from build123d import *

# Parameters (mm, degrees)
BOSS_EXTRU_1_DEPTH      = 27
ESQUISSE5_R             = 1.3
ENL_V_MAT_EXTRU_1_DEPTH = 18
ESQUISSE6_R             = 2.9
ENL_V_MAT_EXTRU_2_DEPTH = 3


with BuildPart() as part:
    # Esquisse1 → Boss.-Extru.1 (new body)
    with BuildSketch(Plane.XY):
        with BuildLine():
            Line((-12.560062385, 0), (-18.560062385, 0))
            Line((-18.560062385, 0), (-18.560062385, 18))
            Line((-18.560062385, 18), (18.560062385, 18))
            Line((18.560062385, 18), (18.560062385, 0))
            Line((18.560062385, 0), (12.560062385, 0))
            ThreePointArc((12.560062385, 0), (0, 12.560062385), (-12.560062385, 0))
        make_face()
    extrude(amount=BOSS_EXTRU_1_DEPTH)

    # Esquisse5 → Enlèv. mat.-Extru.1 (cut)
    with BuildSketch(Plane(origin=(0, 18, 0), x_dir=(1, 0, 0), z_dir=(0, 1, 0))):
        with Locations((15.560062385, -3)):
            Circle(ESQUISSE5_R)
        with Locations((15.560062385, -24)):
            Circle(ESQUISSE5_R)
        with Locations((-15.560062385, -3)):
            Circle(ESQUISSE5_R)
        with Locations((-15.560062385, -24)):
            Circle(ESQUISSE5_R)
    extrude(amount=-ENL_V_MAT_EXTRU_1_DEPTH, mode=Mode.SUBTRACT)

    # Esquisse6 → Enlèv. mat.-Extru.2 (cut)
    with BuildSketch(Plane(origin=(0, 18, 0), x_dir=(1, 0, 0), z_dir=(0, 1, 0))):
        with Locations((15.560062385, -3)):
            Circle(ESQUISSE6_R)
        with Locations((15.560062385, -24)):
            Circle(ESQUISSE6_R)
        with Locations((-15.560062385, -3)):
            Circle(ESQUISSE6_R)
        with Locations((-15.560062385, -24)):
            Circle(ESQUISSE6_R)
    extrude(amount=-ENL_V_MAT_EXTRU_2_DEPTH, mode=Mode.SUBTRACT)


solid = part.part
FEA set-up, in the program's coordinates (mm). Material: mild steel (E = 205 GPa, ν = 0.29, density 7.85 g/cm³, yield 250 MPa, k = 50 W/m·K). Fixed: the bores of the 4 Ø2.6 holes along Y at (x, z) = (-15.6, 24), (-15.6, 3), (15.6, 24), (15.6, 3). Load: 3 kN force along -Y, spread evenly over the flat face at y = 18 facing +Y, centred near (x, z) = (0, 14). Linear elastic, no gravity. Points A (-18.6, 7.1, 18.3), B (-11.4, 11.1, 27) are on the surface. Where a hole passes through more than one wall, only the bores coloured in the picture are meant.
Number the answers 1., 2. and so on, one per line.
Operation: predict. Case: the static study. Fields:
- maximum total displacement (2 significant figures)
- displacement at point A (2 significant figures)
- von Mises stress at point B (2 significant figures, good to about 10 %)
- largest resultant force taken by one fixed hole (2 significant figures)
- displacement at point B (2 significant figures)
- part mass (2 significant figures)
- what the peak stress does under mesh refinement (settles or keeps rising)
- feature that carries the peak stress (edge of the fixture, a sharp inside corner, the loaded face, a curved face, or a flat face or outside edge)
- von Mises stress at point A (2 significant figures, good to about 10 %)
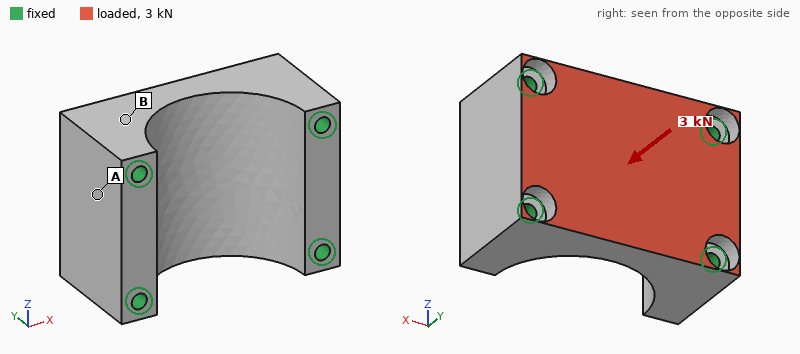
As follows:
1. 1.4 µm
2. 0.26 µm
3. 9.0 MPa
4. 870 N
5. 0.31 µm
6. 84 g
7. keeps rising
8. edge of the fixture
9. 3.1 MPa
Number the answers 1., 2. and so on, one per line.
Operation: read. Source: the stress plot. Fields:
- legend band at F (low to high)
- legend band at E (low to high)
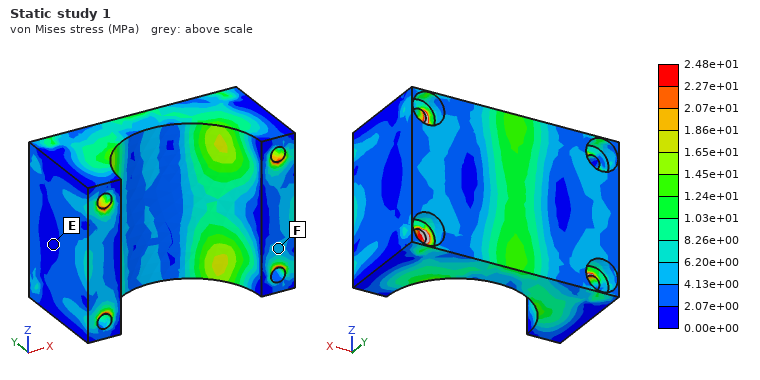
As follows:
1. 4.13e+00 to 6.20e+00 MPa
2. 0.00e+00 to 2.07e+00 MPa
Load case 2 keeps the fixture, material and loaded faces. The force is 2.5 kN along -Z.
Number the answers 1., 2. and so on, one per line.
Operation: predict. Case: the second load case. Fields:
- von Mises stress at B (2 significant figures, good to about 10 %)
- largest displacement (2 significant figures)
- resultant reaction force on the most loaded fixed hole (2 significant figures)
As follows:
1. 9.7 MPa
2. 1.5 µm
3. 830 N
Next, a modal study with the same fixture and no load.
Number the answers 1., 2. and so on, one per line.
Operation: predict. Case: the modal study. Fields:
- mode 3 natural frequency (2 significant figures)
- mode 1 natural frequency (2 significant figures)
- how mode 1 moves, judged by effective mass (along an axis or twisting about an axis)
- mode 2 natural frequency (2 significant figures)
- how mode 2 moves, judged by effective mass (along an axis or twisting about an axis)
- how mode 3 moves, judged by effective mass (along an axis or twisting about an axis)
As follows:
1. 47 kHz
2. 37 kHz
3. along Y
4. 45 kHz
5. along Z
6. along X
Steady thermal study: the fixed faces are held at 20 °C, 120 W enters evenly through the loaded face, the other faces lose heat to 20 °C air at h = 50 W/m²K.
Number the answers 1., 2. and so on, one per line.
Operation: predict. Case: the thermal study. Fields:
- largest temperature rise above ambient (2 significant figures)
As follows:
1. 60 K
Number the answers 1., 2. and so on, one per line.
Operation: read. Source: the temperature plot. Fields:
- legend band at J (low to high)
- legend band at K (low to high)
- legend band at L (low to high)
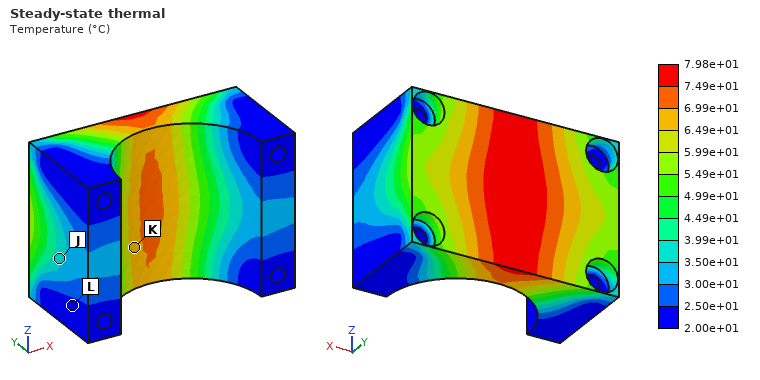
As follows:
1. 3.50e+01 to 3.99e+01 °C
2. 6.49e+01 to 6.99e+01 °C
3. 2.00e+01 to 2.50e+01 °C
